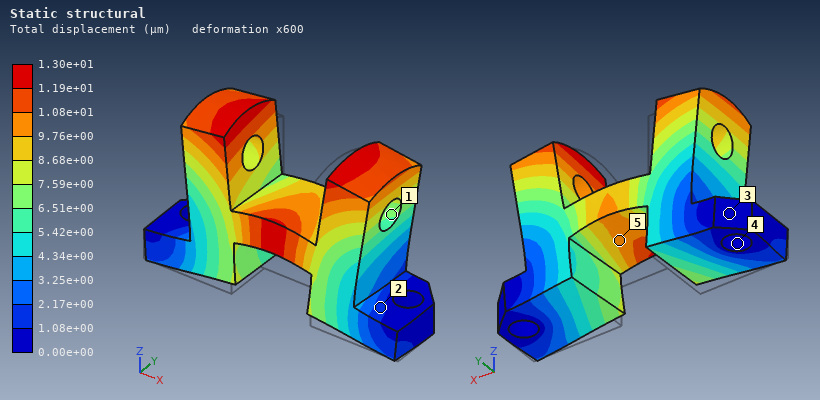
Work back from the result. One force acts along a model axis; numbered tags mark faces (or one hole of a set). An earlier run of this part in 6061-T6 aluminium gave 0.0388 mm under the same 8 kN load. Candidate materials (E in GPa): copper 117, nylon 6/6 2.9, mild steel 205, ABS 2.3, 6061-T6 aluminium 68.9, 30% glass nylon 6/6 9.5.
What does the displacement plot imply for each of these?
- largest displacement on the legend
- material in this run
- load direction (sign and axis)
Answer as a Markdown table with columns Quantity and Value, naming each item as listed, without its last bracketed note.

| Quantity | Value |
|---|---|
| largest displacement on the legend | 1.30e+01 µm |
| material in this run | mild steel |
| load direction | +Z |
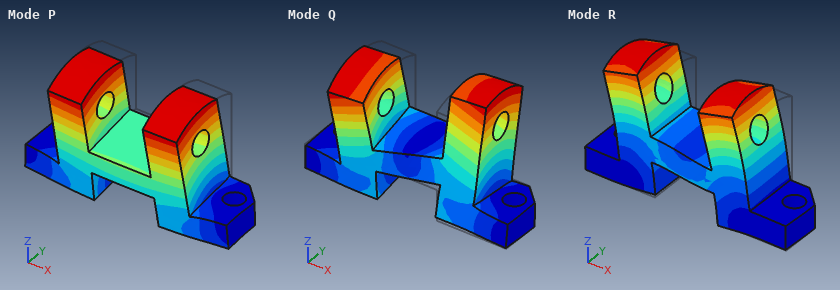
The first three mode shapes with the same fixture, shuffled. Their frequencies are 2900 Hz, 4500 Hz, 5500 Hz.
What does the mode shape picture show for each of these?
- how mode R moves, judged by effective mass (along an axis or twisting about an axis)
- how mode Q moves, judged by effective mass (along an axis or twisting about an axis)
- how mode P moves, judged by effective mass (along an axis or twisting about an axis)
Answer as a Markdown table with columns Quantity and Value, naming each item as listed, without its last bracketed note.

| Quantity | Value |
|---|---|
| how mode R moves, judged by effective mass | along X |
| how mode Q moves, judged by effective mass | twisting about Z |
| how mode P moves, judged by effective mass | along Y |
